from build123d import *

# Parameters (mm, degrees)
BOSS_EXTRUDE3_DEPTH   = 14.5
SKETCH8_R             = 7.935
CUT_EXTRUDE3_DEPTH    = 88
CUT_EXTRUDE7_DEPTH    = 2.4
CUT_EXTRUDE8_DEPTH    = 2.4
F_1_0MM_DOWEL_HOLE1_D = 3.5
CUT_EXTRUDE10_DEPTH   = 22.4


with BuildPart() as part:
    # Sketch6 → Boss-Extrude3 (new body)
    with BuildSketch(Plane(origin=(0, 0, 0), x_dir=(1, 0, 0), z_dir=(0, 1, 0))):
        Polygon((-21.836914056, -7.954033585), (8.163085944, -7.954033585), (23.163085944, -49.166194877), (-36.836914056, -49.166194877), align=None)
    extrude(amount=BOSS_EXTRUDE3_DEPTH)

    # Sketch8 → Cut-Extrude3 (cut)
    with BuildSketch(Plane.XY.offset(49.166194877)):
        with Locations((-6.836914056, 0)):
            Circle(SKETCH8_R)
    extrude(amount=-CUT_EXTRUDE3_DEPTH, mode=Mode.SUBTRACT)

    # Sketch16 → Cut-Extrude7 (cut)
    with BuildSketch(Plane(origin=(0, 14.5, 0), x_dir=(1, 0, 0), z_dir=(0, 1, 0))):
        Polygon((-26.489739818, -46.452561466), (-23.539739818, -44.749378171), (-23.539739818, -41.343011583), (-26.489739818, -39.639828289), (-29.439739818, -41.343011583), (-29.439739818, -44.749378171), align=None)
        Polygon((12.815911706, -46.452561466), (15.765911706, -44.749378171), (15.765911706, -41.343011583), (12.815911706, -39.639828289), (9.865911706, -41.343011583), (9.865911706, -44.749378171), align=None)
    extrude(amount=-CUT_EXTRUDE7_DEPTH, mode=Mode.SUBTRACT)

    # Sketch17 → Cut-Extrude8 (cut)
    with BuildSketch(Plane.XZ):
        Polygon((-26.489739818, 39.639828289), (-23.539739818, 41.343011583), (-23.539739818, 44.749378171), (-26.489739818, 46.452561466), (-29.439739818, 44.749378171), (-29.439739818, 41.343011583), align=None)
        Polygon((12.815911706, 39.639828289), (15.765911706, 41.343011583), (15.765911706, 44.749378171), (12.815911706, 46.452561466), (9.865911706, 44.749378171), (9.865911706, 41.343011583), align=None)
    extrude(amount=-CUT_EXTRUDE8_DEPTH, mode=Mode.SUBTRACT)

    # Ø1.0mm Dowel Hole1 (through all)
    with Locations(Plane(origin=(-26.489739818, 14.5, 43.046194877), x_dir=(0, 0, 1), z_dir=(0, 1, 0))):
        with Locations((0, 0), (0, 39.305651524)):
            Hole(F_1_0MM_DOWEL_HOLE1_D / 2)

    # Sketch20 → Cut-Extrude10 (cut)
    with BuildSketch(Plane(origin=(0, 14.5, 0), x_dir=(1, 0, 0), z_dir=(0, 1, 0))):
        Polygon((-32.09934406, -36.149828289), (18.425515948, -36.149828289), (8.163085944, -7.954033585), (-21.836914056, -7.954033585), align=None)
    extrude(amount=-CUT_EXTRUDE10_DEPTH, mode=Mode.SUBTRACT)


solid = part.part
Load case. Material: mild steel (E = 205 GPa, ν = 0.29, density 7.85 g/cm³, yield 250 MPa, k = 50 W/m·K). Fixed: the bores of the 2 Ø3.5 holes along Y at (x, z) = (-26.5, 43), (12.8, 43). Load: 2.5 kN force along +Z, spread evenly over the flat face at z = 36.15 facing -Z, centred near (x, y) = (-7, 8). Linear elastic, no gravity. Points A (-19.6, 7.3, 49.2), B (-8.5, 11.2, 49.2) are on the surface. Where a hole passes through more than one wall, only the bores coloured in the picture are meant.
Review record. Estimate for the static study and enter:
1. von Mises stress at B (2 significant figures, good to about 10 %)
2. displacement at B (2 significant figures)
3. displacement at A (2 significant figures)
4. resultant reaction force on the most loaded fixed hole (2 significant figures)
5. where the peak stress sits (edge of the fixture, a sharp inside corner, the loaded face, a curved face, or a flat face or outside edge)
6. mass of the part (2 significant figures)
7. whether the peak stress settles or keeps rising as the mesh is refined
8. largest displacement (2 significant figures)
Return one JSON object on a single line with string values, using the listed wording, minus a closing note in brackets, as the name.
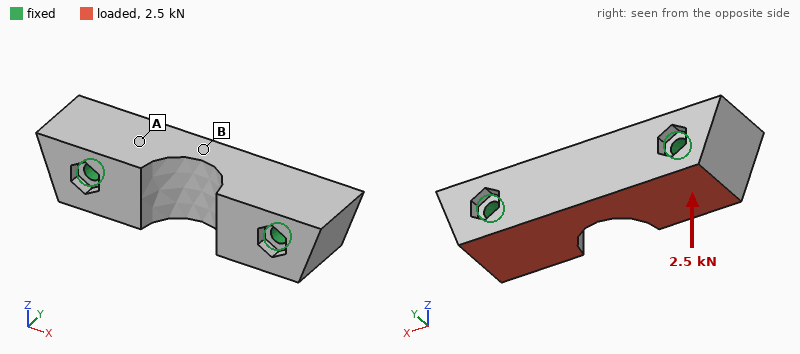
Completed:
{"von Mises stress at B": "17 MPa", "displacement at B": "2.3 µm", "displacement at A": "1.3 µm", "resultant reaction force on the most loaded fixed hole": "1.3 kN", "where the peak stress sits": "edge of the fixture", "mass of the part": "68 g", "whether the peak stress settles or keeps rising as the mesh is refined": "keeps rising", "largest displacement": "2.7 µm"}
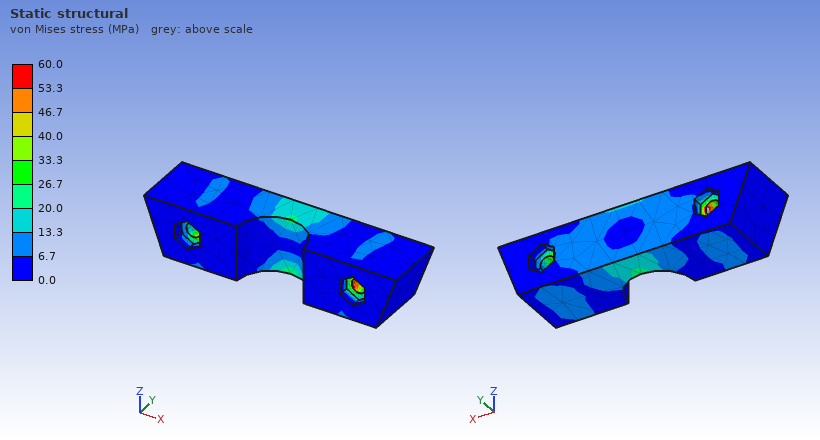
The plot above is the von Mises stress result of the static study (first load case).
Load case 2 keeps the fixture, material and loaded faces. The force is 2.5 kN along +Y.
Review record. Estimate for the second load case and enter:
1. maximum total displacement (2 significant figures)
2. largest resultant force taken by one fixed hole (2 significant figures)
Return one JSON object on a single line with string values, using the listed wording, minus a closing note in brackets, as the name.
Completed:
{"maximum total displacement": "4.4 µm", "largest resultant force taken by one fixed hole": "1.3 kN"}
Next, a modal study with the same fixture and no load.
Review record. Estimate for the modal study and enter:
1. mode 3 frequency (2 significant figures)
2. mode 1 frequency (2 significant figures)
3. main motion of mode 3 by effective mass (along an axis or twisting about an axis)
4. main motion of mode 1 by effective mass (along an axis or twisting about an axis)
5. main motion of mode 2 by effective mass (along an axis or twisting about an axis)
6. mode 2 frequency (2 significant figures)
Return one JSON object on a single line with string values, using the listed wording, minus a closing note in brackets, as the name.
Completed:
{"mode 3 frequency": "36 kHz", "mode 1 frequency": "21 kHz", "main motion of mode 3 by effective mass": "twisting about X", "main motion of mode 1 by effective mass": "along Z", "main motion of mode 2 by effective mass": "along Y", "mode 2 frequency": "25 kHz"}
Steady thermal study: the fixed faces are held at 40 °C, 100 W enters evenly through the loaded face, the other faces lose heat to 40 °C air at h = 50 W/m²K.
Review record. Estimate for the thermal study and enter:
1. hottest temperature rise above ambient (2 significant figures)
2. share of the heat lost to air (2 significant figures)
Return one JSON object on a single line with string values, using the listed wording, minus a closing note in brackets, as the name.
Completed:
{"hottest temperature rise above ambient": "59 K", "share of the heat lost to air": "3.3 %"}
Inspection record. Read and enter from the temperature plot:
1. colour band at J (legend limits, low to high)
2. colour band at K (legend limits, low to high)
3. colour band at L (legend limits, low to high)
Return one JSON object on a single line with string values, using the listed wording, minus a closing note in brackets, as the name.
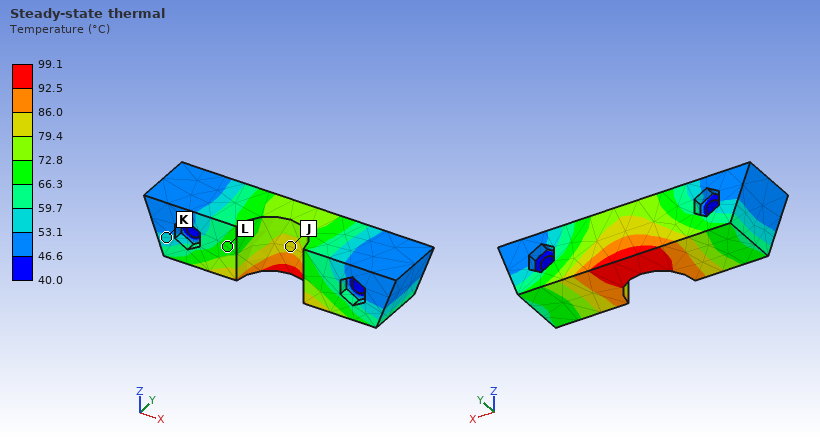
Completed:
{"colour band at J": "79.4 to 86.0 °C", "colour band at K": "53.1 to 59.7 °C", "colour band at L": "66.3 to 72.8 °C"}
